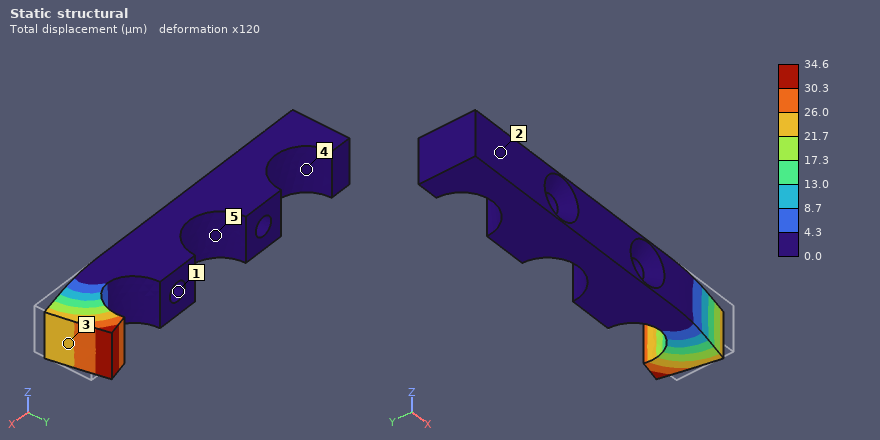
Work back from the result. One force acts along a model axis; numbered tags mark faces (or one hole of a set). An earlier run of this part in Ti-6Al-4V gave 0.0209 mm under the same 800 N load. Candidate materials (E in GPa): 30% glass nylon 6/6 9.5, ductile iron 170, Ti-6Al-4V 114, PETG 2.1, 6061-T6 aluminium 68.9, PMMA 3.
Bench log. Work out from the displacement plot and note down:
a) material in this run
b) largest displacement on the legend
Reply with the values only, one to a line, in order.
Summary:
6061-T6 aluminium
34.6 µm
